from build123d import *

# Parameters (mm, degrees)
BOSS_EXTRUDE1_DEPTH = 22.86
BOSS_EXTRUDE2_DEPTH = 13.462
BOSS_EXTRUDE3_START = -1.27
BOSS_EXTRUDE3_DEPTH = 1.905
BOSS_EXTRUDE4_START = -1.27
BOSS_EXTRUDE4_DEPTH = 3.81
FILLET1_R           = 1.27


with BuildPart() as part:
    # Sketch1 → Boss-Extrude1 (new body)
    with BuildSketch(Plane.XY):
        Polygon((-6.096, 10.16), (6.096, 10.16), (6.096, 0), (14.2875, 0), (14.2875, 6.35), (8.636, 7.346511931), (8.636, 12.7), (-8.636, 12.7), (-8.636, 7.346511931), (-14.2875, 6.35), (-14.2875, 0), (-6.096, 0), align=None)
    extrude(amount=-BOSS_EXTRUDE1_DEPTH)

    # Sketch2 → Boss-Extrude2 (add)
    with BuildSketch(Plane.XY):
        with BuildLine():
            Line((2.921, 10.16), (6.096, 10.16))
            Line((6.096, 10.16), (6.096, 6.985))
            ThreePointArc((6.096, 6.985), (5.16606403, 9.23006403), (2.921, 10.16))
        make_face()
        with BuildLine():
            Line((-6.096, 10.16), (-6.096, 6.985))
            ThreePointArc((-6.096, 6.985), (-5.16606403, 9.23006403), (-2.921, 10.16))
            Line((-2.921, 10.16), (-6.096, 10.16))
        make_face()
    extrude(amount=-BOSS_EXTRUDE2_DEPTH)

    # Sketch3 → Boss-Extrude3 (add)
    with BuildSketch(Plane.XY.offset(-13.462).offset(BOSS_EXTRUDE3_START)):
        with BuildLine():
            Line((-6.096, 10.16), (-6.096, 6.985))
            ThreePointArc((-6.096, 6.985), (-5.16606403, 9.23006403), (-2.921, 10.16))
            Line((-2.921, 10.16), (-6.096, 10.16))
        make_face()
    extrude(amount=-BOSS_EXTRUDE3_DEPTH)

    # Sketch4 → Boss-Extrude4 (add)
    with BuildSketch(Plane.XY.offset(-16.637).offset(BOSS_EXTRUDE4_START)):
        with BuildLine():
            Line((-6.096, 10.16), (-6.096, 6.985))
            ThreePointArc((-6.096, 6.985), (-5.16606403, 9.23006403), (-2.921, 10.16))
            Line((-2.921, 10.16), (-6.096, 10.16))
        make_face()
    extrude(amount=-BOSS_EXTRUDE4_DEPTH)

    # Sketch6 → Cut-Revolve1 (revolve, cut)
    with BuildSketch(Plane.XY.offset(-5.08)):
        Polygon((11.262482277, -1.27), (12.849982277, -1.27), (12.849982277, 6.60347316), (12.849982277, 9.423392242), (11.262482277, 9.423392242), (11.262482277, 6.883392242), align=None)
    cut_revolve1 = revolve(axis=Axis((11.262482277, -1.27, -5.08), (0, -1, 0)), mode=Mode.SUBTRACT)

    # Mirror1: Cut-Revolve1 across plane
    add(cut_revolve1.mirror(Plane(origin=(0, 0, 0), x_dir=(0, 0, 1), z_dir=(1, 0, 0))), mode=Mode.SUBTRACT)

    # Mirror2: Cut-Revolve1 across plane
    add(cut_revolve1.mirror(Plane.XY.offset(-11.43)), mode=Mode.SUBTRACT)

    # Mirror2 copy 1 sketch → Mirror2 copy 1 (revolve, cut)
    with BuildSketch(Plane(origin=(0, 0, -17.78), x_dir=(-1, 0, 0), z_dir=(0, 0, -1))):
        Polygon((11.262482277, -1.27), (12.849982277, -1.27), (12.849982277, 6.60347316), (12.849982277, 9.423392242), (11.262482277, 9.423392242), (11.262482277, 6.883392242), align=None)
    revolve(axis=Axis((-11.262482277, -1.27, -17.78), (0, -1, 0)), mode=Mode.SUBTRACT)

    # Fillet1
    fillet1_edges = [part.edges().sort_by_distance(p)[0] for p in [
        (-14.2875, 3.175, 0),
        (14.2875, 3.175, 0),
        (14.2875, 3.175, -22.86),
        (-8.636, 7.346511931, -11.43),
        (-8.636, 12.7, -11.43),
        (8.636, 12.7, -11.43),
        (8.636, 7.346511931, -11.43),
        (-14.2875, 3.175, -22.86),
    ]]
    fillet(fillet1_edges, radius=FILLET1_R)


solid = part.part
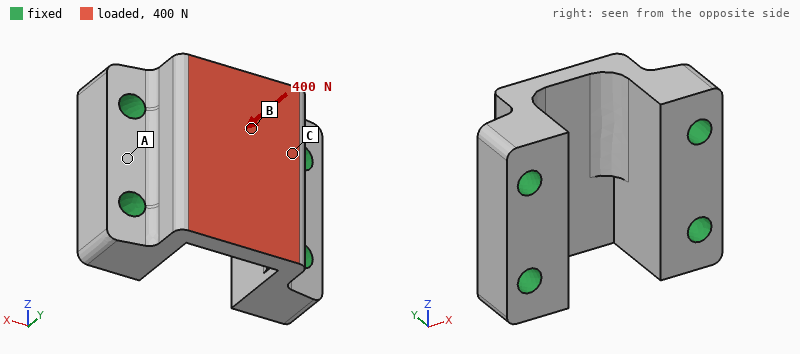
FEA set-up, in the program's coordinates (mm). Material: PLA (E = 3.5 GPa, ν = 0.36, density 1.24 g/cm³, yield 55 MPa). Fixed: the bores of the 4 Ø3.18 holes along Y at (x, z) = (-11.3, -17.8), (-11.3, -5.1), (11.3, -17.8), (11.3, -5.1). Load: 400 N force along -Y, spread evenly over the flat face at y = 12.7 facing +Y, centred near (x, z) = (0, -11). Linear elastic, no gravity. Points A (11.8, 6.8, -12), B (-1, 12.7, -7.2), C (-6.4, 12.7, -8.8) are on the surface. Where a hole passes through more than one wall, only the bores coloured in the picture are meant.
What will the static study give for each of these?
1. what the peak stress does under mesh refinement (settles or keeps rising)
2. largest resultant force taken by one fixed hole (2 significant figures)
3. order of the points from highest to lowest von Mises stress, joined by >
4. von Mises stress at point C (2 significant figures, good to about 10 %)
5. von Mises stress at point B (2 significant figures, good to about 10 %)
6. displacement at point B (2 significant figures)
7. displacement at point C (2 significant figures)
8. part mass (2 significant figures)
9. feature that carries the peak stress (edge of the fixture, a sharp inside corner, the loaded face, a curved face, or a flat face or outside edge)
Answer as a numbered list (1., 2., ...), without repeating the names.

1. keeps rising
2. 130 N
3. B > C > A
4. 2.3 MPa
5. 7.6 MPa
6. 29 µm
7. 13 µm
8. 4.7 g
9. a sharp inside corner
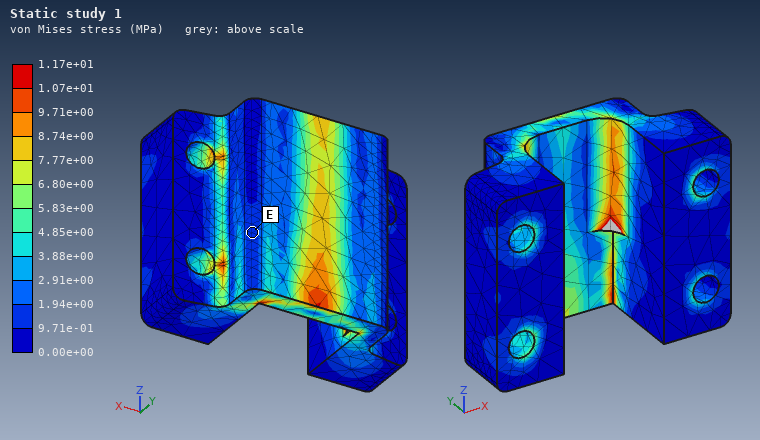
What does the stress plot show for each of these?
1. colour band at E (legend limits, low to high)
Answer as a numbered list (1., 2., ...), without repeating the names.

1. 9.71e-01 to 1.94e+00 MPa
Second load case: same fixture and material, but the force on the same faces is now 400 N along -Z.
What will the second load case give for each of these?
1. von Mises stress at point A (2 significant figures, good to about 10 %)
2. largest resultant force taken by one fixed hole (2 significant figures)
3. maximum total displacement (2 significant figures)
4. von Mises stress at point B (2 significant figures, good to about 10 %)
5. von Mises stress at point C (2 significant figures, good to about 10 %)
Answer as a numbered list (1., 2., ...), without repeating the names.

1. 1.8 MPa
2. 160 N
3. 51 µm
4. 3.1 MPa
5. 4.6 MPa
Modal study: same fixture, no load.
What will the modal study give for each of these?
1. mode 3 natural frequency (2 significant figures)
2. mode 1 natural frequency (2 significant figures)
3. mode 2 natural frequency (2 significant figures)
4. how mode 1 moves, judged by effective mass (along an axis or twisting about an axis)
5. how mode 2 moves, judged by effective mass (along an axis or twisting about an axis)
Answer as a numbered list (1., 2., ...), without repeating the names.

1. 17 kHz
2. 13 kHz
3. 15 kHz
4. along X
5. along Z
